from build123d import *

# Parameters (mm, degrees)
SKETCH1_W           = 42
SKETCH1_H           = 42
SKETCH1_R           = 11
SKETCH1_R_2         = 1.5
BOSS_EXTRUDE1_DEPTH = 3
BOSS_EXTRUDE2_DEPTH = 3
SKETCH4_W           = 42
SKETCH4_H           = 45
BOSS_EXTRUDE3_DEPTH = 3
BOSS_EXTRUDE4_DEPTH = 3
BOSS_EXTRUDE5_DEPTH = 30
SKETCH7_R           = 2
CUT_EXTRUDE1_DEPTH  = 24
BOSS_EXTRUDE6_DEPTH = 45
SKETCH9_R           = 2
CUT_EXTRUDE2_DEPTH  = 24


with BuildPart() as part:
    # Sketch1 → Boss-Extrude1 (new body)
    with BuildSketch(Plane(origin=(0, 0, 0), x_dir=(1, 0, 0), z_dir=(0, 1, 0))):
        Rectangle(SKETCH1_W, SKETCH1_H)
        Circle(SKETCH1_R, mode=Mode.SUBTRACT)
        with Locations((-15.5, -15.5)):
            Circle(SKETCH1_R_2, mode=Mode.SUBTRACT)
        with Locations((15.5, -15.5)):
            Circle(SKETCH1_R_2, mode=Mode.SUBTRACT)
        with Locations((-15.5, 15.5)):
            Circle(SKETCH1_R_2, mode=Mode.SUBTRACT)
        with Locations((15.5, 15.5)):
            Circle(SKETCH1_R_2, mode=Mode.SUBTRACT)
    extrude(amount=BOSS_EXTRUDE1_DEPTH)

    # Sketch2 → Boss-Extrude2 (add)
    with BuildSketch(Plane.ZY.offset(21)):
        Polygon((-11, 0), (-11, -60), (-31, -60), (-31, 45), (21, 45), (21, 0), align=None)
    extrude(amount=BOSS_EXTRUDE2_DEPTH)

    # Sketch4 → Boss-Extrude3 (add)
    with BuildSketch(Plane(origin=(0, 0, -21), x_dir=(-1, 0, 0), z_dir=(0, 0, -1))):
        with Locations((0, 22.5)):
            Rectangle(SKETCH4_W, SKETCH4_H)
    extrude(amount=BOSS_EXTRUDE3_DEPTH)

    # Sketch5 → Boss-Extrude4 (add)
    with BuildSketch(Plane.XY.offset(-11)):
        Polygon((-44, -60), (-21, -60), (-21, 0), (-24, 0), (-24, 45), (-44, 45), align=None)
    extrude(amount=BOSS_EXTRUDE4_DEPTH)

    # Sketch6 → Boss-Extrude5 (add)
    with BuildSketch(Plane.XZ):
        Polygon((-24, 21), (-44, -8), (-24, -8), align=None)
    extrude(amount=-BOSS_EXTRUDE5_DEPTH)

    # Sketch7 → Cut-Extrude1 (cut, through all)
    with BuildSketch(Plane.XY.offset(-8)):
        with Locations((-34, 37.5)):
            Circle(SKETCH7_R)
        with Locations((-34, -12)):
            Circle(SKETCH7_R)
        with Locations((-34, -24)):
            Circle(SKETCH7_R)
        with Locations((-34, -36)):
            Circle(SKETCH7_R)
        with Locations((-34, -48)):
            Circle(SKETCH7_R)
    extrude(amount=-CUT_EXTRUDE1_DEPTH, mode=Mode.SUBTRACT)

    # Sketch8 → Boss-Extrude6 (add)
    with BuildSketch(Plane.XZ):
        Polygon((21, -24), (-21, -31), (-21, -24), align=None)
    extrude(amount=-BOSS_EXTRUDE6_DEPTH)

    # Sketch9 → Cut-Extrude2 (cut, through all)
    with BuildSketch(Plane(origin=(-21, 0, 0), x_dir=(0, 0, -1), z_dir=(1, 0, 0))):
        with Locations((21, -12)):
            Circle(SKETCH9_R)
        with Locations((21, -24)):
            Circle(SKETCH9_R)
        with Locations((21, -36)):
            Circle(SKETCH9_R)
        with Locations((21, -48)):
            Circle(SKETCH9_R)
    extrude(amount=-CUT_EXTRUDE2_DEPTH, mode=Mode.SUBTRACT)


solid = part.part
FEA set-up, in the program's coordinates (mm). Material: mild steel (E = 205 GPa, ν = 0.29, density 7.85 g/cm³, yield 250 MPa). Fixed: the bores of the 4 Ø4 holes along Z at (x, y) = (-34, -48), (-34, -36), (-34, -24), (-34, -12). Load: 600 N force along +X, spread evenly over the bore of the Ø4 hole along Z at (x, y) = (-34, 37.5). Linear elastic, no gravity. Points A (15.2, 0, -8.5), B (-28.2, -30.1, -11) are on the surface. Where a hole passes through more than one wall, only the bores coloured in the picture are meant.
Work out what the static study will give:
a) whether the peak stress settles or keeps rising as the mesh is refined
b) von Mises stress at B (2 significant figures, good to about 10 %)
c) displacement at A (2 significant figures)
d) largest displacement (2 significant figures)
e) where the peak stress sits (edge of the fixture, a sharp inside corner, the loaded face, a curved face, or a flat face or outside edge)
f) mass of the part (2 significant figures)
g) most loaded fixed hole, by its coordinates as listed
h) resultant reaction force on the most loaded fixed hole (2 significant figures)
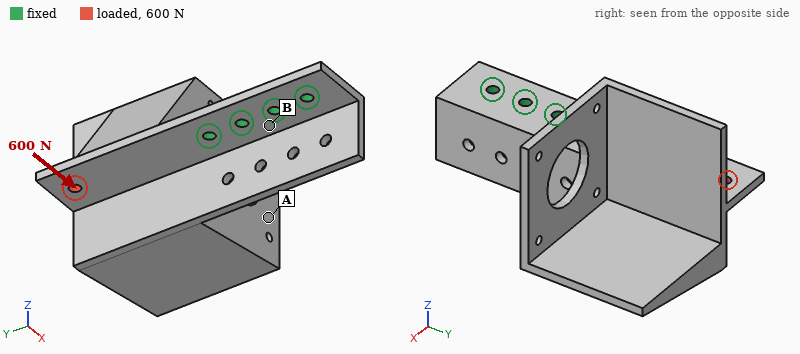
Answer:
keeps rising
25 MPa
50 µm
82 µm
edge of the fixture
330 g
(-34, -12)
1.8 kN
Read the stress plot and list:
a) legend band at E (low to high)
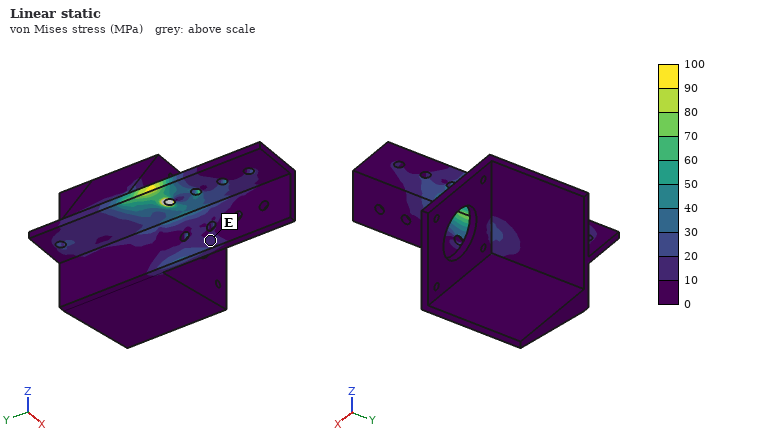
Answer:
10 to 20 MPa
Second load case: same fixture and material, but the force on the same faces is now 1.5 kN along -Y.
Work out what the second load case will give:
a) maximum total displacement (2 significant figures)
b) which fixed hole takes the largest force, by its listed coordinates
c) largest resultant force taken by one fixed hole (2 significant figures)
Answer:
9.1 µm
(-34, -12)
1.1 kN
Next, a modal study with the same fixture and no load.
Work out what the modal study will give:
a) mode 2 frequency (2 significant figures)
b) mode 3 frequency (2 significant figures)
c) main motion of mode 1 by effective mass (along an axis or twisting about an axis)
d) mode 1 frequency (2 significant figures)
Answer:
1300 Hz
1400 Hz
along Z
510 Hz
